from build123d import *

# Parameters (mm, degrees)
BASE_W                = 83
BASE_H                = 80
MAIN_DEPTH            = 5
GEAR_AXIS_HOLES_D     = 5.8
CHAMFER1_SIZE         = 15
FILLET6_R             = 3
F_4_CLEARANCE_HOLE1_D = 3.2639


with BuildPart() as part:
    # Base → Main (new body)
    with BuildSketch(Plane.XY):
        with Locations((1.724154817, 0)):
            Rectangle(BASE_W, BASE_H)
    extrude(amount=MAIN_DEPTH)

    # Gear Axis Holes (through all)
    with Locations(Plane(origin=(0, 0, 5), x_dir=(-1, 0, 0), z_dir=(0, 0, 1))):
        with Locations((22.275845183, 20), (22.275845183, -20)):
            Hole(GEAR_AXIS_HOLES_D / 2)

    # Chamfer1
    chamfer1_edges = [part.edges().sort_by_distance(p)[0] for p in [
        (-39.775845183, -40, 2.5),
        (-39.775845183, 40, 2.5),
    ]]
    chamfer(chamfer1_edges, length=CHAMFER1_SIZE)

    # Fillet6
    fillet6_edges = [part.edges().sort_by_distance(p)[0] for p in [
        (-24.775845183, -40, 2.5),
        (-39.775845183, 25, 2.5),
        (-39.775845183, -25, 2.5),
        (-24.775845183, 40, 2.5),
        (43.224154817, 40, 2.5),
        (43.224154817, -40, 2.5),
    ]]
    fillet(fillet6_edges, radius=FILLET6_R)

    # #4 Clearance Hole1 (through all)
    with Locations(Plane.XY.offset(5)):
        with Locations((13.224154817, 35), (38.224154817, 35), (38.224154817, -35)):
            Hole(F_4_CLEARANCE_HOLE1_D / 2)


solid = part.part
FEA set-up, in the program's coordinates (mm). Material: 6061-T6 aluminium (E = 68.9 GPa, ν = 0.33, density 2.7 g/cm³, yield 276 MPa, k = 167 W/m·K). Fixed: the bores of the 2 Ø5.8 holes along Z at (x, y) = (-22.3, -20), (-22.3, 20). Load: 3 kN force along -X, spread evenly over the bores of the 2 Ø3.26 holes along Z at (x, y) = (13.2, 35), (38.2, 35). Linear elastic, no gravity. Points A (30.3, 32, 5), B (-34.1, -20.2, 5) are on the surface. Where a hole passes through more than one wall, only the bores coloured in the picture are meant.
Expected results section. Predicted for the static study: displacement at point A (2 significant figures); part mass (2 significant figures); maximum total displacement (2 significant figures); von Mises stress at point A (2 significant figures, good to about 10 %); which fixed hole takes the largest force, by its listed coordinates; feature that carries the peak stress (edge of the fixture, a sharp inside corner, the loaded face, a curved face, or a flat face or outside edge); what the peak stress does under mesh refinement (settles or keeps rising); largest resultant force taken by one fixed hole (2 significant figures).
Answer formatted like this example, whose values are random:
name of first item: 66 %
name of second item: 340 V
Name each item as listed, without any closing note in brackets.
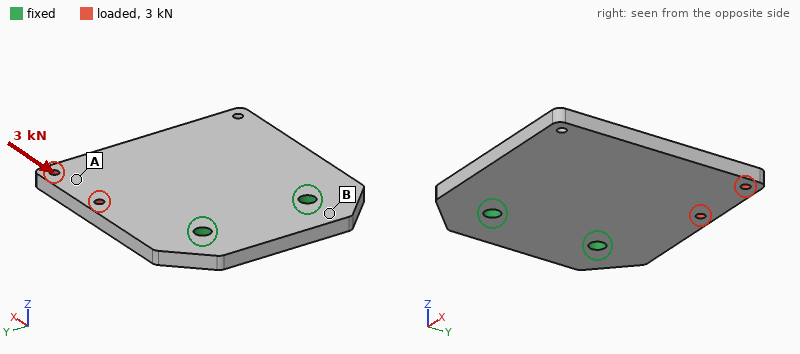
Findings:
displacement at point A: 32 µm
part mass: 85 g
maximum total displacement: 45 µm
von Mises stress at point A: 21 MPa
which fixed hole takes the largest force, by its listed coordinates: (-22.3, 20)
feature that carries the peak stress: edge of the fixture
what the peak stress does under mesh refinement: keeps rising
largest resultant force taken by one fixed hole: 4.0 kN
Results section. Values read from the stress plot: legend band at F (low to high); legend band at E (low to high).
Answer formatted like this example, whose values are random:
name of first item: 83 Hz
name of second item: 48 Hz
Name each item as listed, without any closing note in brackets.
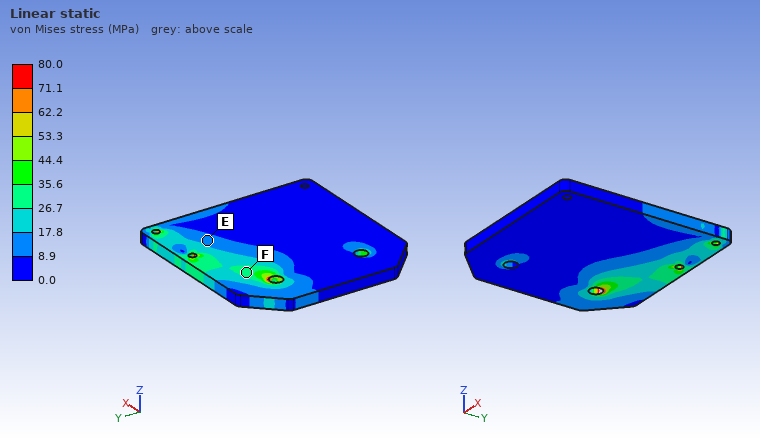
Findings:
legend band at F: 26.7 to 35.6 MPa
legend band at E: 8.9 to 17.8 MPa
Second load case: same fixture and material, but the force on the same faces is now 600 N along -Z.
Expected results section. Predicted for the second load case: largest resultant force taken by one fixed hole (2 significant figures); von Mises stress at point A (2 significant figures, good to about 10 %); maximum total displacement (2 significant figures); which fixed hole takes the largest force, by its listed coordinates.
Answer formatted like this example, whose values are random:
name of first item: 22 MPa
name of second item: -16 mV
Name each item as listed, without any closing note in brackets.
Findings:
largest resultant force taken by one fixed hole: 710 N
von Mises stress at point A: 35 MPa
maximum total displacement: 0.98 mm
which fixed hole takes the largest force, by its listed coordinates: (-22.3, 20)
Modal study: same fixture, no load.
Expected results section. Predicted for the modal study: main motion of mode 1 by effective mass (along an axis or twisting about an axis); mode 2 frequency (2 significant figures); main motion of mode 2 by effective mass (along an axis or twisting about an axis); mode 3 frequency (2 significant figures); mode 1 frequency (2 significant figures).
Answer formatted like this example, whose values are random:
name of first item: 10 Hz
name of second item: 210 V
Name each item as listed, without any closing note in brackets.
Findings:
main motion of mode 1 by effective mass: along Z
mode 2 frequency: 1900 Hz
main motion of mode 2 by effective mass: twisting about X
mode 3 frequency: 4800 Hz
mode 1 frequency: 940 Hz
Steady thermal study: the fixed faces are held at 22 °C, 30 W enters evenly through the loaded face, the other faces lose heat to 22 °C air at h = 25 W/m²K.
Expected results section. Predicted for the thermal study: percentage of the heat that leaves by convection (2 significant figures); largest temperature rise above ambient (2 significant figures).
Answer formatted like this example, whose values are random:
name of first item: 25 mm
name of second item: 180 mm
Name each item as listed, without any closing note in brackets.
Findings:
percentage of the heat that leaves by convection: 14 %
largest temperature rise above ambient: 43 K
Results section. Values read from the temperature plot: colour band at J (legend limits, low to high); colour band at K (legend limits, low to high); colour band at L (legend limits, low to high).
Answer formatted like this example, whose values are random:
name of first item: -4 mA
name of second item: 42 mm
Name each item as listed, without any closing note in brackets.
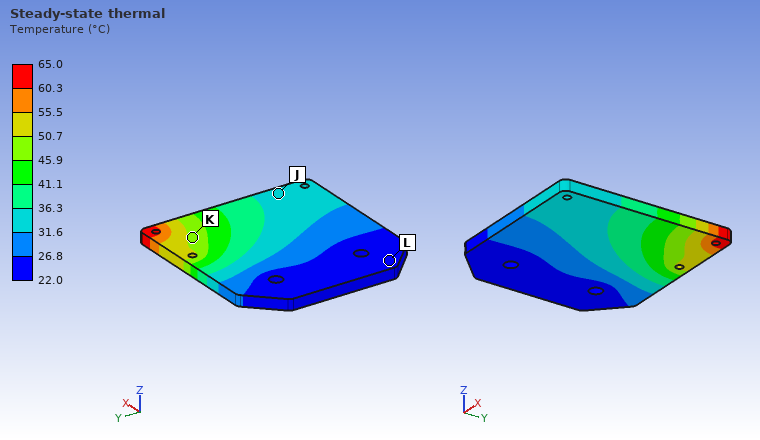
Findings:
colour band at J: 31.6 to 36.3 °C
colour band at K: 45.9 to 50.7 °C
colour band at L: 22.0 to 26.8 °C
